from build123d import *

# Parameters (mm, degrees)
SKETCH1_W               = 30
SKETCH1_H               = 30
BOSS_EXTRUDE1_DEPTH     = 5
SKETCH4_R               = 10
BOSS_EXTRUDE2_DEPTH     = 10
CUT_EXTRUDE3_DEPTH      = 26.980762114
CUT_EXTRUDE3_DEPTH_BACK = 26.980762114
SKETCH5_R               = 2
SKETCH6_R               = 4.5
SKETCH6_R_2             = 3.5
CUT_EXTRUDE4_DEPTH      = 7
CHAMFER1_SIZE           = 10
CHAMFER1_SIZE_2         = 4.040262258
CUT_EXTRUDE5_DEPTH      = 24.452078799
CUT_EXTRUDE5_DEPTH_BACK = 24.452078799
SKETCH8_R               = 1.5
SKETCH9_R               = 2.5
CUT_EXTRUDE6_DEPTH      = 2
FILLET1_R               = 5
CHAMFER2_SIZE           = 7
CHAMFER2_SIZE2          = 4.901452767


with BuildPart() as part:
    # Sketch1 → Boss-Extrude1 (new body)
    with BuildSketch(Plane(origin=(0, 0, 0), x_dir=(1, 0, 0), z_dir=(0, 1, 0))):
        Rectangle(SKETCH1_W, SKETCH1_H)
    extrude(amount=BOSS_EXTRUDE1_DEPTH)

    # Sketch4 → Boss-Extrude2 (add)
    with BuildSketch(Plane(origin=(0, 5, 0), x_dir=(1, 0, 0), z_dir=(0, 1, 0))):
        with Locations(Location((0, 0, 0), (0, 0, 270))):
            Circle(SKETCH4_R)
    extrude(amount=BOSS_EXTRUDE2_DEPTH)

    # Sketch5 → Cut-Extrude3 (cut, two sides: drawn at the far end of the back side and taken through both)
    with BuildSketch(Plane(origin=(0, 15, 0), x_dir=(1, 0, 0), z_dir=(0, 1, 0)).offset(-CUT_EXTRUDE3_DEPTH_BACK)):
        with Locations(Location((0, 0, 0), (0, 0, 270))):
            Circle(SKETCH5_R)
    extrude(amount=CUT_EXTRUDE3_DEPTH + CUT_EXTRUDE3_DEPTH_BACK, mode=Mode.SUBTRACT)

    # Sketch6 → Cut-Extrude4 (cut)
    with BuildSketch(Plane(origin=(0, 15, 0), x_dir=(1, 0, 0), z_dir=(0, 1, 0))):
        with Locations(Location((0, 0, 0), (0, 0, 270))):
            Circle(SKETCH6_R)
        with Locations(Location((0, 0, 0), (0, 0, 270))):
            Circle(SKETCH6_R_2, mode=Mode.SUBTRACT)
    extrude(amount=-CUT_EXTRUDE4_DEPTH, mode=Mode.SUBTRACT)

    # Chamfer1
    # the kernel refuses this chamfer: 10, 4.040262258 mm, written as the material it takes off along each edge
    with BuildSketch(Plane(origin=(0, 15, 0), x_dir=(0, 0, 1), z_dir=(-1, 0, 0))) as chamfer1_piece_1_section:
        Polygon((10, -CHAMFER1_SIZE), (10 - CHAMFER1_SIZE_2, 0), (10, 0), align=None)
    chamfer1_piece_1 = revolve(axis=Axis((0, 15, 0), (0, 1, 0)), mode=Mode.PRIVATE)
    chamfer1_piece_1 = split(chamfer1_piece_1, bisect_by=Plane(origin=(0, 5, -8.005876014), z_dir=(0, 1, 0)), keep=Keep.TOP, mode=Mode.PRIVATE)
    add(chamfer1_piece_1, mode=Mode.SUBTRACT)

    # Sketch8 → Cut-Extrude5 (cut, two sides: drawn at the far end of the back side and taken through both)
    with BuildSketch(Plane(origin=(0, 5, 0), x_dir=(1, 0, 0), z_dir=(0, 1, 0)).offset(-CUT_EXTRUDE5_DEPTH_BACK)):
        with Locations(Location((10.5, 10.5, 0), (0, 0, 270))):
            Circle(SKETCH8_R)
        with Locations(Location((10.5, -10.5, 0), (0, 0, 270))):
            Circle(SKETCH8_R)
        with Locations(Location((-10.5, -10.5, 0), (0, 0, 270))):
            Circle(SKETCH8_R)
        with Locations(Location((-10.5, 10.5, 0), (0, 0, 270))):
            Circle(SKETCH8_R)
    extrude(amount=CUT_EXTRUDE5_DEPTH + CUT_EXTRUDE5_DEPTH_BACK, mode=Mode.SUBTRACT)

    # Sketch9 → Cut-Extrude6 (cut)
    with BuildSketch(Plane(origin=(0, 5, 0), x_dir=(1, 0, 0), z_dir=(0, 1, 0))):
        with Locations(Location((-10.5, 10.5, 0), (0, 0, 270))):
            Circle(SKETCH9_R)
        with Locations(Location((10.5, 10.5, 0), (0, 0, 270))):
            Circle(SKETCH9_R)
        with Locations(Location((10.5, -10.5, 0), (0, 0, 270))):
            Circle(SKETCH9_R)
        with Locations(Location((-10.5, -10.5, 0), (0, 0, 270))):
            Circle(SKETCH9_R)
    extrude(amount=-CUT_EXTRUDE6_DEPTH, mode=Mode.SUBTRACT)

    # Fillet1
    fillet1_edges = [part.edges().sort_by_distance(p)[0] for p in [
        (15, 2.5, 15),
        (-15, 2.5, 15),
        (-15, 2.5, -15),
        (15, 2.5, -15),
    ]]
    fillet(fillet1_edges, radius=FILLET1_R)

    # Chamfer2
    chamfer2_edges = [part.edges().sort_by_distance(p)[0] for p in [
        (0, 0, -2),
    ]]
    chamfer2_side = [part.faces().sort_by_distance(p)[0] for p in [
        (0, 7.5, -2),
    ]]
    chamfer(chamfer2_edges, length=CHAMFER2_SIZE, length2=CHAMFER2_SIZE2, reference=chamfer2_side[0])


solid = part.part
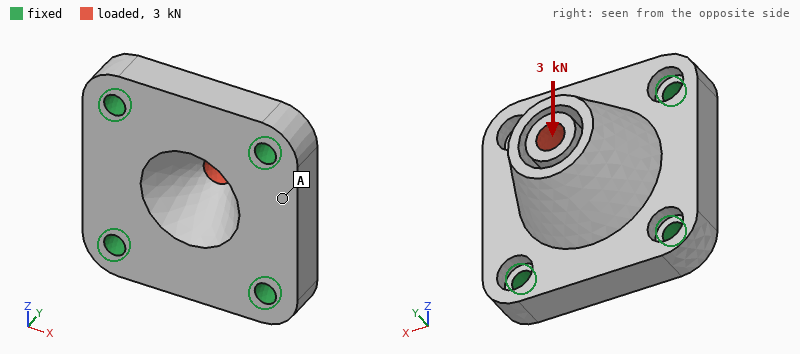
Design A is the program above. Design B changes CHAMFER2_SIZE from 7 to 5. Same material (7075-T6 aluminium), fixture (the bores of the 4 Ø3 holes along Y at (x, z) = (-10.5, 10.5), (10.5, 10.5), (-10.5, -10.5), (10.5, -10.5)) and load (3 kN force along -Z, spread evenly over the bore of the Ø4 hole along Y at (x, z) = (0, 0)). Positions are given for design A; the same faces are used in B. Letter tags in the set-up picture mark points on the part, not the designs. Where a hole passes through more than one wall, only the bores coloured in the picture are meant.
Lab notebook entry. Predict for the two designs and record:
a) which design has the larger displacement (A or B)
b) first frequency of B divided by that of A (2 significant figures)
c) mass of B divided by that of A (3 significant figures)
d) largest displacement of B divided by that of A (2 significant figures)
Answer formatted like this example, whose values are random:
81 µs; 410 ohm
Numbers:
A; 0.98; 1.02; 0.79
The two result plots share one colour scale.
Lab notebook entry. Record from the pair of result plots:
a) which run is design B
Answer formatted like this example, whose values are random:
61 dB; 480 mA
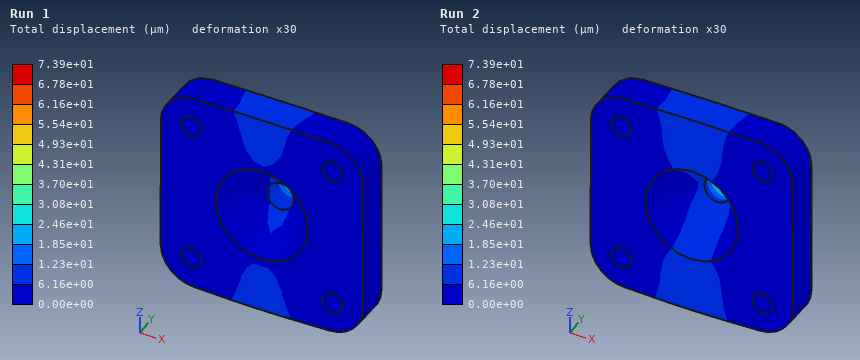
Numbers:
Run 1
